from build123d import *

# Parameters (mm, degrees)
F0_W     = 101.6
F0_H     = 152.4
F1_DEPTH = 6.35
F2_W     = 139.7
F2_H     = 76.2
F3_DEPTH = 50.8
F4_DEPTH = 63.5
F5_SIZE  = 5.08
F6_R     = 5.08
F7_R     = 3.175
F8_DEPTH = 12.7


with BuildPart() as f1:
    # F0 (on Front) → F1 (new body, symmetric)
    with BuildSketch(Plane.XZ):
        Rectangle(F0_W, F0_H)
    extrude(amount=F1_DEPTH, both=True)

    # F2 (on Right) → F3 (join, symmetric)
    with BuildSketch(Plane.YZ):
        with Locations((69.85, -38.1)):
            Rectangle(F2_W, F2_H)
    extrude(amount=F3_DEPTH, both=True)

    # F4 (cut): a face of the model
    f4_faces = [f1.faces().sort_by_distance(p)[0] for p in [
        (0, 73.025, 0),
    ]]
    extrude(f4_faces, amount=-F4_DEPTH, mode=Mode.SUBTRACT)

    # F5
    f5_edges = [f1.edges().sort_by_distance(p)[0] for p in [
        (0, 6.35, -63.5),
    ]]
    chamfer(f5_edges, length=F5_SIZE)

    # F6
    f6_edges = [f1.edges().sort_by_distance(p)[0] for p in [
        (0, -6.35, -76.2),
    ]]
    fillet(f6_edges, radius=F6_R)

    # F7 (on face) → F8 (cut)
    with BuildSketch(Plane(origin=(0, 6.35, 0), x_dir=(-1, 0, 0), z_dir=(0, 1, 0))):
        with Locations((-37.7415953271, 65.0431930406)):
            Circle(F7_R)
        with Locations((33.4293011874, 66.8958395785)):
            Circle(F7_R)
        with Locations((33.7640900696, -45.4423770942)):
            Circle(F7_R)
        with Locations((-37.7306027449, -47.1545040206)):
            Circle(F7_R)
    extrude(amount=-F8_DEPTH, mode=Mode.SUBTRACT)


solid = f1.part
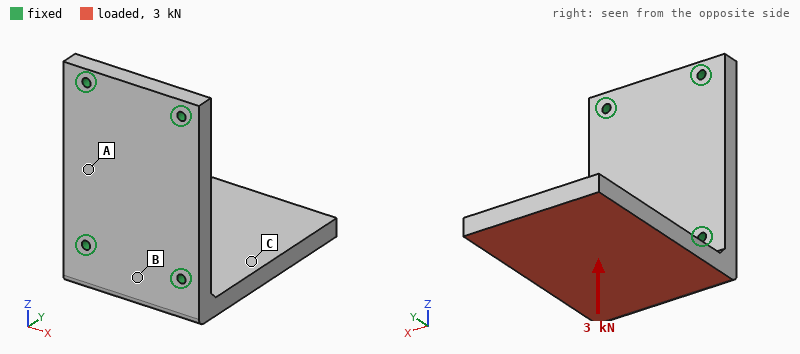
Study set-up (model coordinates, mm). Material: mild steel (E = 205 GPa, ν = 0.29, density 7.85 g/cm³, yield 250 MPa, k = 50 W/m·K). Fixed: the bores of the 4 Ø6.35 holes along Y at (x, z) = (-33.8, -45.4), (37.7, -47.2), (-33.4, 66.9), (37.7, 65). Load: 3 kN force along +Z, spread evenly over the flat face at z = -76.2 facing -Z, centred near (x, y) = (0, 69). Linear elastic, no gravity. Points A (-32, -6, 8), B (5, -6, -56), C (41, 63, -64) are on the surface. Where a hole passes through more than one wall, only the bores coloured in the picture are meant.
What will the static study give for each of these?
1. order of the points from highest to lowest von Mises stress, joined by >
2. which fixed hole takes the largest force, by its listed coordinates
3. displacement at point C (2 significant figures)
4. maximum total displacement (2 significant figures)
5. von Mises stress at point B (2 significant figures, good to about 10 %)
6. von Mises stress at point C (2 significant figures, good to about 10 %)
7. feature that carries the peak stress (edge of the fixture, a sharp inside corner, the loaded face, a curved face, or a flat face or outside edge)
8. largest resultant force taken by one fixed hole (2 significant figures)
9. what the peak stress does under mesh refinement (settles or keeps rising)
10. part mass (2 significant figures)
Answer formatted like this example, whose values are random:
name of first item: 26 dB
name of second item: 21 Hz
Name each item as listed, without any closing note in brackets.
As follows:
order of the points from highest to lowest von Mises stress, joined by >: B > C > A
which fixed hole takes the largest force, by its listed coordinates: (-33.8, -45.4)
displacement at point C: 0.15 mm
maximum total displacement: 0.42 mm
von Mises stress at point B: 51 MPa
von Mises stress at point C: 23 MPa
feature that carries the peak stress: edge of the fixture
largest resultant force taken by one fixed hole: 1.4 kN
what the peak stress does under mesh refinement: keeps rising
part mass: 2.9 kg
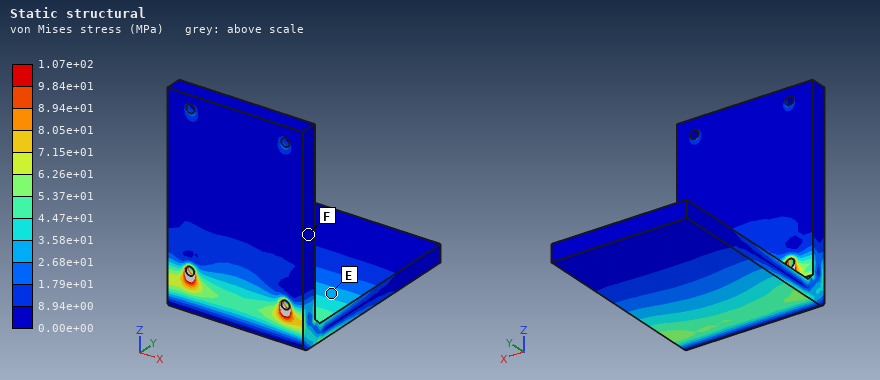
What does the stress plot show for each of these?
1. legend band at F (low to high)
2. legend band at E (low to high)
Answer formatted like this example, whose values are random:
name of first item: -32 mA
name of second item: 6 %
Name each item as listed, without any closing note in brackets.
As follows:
legend band at F: 0.00e+00 to 8.94e+00 MPa
legend band at E: 2.68e+01 to 3.58e+01 MPa
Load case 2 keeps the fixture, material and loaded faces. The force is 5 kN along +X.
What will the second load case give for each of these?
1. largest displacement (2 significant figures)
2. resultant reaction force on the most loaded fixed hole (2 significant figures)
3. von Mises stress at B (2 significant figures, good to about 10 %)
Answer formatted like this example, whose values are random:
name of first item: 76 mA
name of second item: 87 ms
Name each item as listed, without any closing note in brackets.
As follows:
largest displacement: 53 µm
resultant reaction force on the most loaded fixed hole: 5.6 kN
von Mises stress at B: 12 MPa
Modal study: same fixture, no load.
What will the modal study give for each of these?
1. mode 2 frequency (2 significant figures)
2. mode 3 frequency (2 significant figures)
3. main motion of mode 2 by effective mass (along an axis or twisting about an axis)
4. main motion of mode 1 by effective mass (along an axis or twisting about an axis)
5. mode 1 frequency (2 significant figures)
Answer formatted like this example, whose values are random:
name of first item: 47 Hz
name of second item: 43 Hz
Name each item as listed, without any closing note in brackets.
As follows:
mode 2 frequency: 1300 Hz
mode 3 frequency: 1800 Hz
main motion of mode 2 by effective mass: along X
main motion of mode 1 by effective mass: along Z
mode 1 frequency: 440 Hz
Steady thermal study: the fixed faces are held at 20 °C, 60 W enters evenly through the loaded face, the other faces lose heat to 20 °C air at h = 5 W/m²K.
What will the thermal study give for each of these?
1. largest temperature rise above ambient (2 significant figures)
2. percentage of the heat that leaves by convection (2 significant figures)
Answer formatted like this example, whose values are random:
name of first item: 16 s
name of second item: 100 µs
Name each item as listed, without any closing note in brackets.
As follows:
largest temperature rise above ambient: 77 K
percentage of the heat that leaves by convection: 11 %
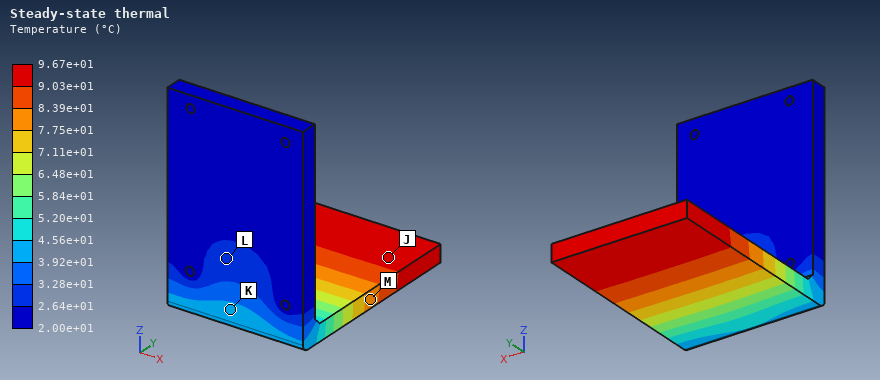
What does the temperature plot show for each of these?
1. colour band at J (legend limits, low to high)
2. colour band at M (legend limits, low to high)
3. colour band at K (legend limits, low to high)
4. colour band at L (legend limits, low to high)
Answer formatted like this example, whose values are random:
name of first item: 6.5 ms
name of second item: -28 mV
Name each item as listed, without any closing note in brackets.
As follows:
colour band at J: 9.03e+01 to 9.67e+01 °C
colour band at M: 7.75e+01 to 8.39e+01 °C
colour band at K: 3.92e+01 to 4.56e+01 °C
colour band at L: 2.64e+01 to 3.28e+01 °C
